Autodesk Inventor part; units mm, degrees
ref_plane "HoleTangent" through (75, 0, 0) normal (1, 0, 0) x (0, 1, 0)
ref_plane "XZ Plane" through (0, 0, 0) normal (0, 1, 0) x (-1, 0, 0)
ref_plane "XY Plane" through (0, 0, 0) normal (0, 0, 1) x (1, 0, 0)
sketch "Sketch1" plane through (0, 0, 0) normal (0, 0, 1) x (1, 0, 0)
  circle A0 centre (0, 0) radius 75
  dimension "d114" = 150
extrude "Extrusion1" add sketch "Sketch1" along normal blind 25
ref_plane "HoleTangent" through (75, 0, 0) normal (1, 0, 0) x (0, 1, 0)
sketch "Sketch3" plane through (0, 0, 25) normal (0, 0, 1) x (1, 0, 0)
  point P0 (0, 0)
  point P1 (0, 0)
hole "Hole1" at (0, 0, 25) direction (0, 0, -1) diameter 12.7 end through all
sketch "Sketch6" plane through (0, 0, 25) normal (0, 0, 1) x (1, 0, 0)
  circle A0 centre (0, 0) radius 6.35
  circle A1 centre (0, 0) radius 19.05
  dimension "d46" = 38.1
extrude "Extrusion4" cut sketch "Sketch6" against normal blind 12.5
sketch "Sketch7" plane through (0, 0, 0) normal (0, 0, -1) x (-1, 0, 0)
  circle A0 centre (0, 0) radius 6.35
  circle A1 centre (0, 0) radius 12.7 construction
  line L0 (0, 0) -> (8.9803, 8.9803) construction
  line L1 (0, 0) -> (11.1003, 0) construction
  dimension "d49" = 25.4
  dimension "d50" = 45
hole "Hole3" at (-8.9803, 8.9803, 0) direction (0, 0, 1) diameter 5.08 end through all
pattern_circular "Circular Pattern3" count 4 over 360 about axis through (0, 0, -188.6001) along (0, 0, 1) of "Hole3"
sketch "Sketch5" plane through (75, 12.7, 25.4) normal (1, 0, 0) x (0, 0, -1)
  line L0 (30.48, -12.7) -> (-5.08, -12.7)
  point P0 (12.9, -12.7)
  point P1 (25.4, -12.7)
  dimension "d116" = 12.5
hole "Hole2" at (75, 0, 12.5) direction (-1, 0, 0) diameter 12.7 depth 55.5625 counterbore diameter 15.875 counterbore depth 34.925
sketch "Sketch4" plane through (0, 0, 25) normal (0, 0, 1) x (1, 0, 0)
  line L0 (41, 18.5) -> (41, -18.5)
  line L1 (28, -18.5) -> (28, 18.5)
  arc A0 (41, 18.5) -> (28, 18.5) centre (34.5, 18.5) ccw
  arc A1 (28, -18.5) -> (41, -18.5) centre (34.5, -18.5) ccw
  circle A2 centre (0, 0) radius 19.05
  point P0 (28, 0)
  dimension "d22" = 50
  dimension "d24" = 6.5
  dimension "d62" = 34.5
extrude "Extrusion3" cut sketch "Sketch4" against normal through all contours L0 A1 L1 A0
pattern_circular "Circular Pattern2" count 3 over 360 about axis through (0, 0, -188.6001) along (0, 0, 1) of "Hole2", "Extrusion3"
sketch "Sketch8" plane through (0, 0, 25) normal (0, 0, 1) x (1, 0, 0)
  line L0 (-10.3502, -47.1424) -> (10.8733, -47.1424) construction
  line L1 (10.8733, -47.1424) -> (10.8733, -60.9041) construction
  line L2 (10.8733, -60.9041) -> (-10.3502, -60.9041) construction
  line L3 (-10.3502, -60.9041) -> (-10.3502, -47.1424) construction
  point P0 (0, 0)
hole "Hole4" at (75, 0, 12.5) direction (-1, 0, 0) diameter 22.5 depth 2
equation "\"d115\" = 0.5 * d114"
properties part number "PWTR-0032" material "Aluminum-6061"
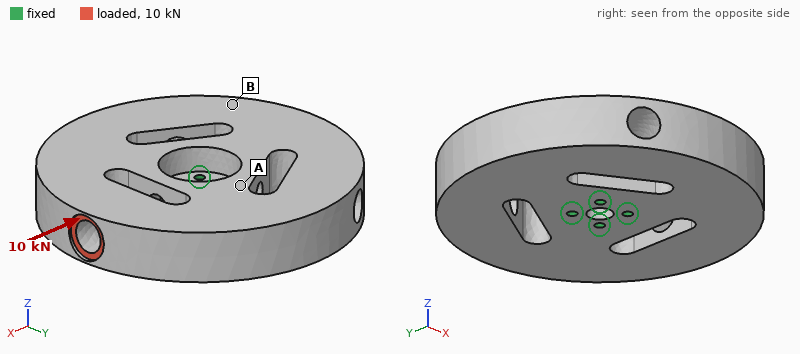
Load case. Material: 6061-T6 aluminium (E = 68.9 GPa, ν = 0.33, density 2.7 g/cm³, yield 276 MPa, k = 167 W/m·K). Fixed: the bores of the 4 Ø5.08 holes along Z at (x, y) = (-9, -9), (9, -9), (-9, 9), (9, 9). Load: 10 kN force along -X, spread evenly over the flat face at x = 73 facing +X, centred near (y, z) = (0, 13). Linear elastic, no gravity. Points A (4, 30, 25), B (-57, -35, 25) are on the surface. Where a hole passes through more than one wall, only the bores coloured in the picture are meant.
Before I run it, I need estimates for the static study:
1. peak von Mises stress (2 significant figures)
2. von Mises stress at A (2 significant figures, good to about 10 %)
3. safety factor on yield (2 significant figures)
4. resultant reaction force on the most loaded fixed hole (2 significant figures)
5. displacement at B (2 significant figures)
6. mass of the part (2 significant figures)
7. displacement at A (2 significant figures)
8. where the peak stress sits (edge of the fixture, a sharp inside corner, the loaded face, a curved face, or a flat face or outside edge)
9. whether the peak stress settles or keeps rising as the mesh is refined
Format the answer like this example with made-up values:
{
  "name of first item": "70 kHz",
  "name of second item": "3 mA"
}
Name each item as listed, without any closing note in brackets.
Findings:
{
  "peak von Mises stress": "100 MPa",
  "von Mises stress at A": "8.5 MPa",
  "safety factor on yield": "2.8",
  "resultant reaction force on the most loaded fixed hole": "3.0 kN",
  "displacement at B": "21 µm",
  "mass of the part": "960 g",
  "displacement at A": "12 µm",
  "where the peak stress sits": "the loaded face",
  "whether the peak stress settles or keeps rising as the mesh is refined": "settles"
}
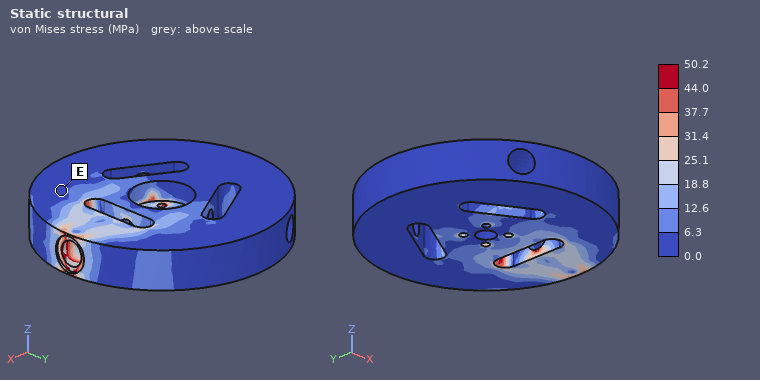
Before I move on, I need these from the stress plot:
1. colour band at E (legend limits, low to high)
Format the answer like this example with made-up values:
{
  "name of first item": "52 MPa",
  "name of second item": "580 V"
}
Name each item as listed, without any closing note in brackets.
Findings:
{
  "colour band at E": "0.0 to 6.3 MPa"
}
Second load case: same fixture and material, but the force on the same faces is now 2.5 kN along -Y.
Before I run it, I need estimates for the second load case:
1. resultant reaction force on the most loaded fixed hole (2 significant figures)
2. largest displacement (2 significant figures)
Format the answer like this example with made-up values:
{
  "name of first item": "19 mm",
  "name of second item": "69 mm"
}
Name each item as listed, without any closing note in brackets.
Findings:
{
  "resultant reaction force on the most loaded fixed hole": "3.6 kN",
  "largest displacement": "30 µm"
}
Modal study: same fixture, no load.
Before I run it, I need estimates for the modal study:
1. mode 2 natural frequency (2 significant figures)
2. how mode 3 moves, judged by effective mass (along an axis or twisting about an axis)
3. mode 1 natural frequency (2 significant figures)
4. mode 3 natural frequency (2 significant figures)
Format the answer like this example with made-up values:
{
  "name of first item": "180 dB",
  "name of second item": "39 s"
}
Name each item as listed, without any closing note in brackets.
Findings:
{
  "mode 2 natural frequency": "1700 Hz",
  "how mode 3 moves, judged by effective mass": "twisting about Z",
  "mode 1 natural frequency": "1700 Hz",
  "mode 3 natural frequency": "2300 Hz"
}
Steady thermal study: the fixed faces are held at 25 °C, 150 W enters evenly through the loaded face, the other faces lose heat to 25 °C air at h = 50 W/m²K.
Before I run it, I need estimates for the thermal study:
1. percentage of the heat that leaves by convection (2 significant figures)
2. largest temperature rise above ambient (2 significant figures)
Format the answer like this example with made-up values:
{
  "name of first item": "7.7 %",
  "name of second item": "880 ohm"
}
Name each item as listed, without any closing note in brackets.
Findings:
{
  "percentage of the heat that leaves by convection": "28 %",
  "largest temperature rise above ambient": "66 K"
}
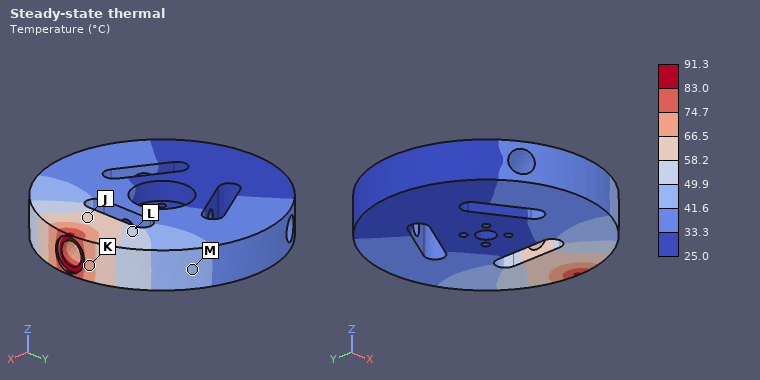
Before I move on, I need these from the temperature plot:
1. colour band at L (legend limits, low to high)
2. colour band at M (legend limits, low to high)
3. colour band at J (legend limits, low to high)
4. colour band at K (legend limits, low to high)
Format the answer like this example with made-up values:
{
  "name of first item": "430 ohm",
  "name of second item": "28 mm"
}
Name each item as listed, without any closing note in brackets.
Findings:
{
  "colour band at L": "49.9 to 58.2 °C",
  "colour band at M": "41.6 to 49.9 °C",
  "colour band at J": "58.2 to 66.5 °C",
  "colour band at K": "66.5 to 74.7 °C"
}
